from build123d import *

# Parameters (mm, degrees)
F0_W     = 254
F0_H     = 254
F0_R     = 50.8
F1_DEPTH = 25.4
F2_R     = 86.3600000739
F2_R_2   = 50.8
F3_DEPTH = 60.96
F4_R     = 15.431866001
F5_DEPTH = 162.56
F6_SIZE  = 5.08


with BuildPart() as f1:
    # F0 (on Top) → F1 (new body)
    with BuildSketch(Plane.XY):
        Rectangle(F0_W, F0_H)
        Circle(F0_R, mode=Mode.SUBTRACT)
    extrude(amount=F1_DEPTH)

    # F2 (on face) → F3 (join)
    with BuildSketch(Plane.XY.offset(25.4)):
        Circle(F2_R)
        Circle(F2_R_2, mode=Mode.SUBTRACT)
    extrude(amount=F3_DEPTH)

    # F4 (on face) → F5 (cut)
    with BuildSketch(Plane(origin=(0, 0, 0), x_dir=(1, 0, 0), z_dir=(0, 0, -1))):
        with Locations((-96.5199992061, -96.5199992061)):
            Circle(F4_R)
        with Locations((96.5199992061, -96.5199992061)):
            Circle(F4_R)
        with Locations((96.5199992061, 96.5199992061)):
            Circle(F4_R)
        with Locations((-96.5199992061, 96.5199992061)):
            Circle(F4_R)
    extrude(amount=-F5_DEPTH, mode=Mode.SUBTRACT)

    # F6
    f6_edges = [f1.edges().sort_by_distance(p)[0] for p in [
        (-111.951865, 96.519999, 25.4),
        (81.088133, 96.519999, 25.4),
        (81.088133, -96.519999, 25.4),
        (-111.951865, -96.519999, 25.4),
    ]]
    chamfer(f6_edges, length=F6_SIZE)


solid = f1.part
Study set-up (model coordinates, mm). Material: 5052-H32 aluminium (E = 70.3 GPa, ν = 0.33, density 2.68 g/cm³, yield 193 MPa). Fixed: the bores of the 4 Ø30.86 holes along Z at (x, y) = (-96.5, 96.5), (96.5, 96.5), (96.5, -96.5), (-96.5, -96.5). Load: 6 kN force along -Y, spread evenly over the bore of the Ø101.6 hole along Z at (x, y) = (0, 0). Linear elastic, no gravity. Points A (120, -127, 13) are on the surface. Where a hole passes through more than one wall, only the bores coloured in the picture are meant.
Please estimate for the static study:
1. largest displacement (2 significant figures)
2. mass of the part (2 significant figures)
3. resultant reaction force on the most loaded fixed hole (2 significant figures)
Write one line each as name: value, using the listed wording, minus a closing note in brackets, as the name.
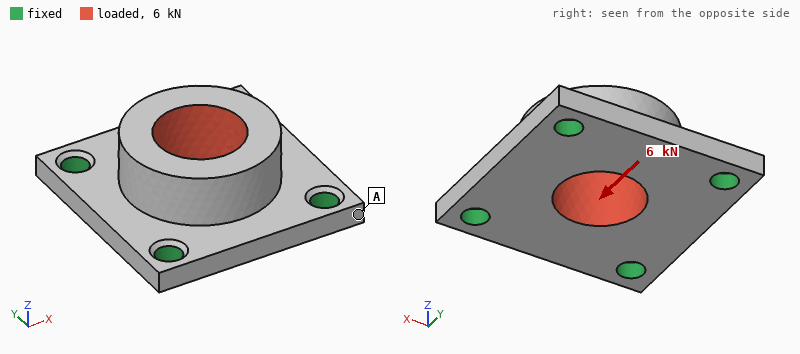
largest displacement: 3.4 µm
mass of the part: 6.1 kg
resultant reaction force on the most loaded fixed hole: 1.7 kN
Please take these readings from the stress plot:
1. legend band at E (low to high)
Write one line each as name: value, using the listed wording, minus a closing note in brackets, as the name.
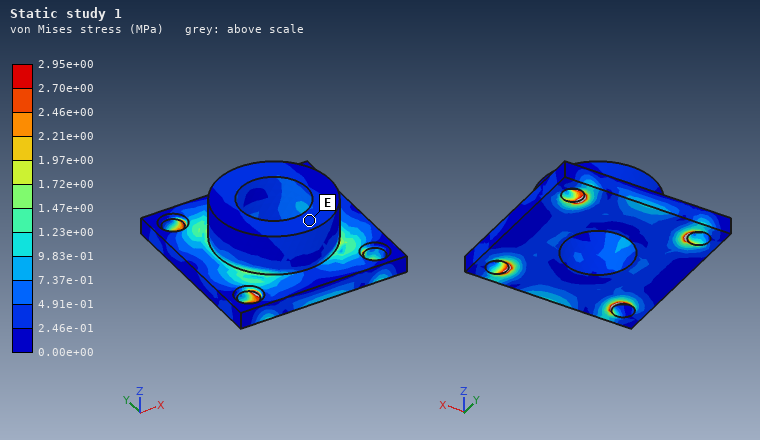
legend band at E: 2.46e-01 to 4.91e-01 MPa
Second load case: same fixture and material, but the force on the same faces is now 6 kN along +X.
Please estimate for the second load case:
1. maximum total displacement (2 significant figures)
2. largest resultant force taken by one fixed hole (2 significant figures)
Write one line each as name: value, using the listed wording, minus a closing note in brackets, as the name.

maximum total displacement: 3.5 µm
largest resultant force taken by one fixed hole: 1.7 kN
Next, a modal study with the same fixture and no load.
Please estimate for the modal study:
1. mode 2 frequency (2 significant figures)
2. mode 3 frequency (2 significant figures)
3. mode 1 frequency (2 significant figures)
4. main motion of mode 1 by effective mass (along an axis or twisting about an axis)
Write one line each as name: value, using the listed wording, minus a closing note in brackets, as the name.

mode 2 frequency: 3200 Hz
mode 3 frequency: 3200 Hz
mode 1 frequency: 2700 Hz
main motion of mode 1 by effective mass: along Z
